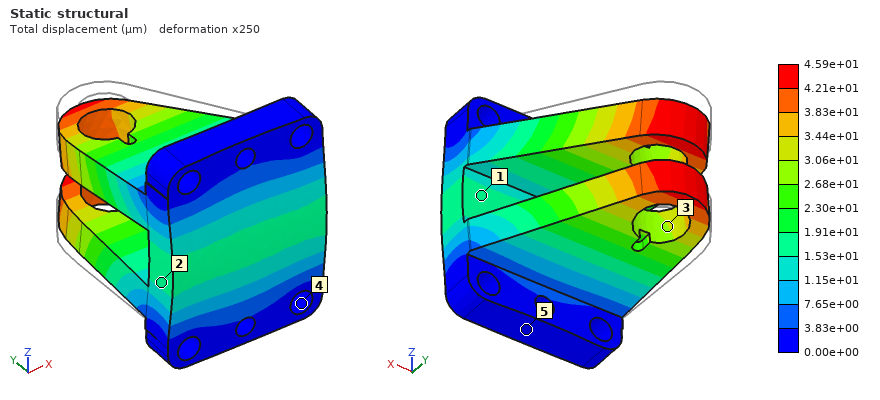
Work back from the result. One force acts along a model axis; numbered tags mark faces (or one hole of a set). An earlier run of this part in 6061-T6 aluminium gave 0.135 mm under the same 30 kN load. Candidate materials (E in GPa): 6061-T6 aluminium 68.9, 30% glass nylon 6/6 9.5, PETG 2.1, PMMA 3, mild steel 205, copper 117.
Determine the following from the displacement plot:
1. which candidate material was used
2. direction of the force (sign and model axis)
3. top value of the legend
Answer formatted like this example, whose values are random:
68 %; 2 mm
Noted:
mild steel; -Y; 4.59e+01 µm
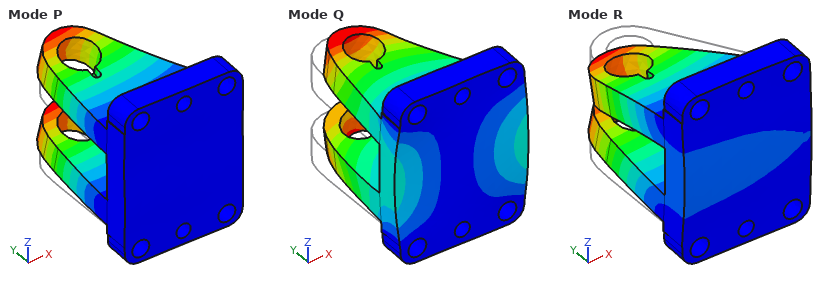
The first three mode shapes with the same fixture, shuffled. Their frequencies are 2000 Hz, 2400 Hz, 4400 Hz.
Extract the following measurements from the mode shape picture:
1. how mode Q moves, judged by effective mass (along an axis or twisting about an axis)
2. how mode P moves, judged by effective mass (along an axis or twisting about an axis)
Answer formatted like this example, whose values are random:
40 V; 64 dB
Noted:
along X; along Z
